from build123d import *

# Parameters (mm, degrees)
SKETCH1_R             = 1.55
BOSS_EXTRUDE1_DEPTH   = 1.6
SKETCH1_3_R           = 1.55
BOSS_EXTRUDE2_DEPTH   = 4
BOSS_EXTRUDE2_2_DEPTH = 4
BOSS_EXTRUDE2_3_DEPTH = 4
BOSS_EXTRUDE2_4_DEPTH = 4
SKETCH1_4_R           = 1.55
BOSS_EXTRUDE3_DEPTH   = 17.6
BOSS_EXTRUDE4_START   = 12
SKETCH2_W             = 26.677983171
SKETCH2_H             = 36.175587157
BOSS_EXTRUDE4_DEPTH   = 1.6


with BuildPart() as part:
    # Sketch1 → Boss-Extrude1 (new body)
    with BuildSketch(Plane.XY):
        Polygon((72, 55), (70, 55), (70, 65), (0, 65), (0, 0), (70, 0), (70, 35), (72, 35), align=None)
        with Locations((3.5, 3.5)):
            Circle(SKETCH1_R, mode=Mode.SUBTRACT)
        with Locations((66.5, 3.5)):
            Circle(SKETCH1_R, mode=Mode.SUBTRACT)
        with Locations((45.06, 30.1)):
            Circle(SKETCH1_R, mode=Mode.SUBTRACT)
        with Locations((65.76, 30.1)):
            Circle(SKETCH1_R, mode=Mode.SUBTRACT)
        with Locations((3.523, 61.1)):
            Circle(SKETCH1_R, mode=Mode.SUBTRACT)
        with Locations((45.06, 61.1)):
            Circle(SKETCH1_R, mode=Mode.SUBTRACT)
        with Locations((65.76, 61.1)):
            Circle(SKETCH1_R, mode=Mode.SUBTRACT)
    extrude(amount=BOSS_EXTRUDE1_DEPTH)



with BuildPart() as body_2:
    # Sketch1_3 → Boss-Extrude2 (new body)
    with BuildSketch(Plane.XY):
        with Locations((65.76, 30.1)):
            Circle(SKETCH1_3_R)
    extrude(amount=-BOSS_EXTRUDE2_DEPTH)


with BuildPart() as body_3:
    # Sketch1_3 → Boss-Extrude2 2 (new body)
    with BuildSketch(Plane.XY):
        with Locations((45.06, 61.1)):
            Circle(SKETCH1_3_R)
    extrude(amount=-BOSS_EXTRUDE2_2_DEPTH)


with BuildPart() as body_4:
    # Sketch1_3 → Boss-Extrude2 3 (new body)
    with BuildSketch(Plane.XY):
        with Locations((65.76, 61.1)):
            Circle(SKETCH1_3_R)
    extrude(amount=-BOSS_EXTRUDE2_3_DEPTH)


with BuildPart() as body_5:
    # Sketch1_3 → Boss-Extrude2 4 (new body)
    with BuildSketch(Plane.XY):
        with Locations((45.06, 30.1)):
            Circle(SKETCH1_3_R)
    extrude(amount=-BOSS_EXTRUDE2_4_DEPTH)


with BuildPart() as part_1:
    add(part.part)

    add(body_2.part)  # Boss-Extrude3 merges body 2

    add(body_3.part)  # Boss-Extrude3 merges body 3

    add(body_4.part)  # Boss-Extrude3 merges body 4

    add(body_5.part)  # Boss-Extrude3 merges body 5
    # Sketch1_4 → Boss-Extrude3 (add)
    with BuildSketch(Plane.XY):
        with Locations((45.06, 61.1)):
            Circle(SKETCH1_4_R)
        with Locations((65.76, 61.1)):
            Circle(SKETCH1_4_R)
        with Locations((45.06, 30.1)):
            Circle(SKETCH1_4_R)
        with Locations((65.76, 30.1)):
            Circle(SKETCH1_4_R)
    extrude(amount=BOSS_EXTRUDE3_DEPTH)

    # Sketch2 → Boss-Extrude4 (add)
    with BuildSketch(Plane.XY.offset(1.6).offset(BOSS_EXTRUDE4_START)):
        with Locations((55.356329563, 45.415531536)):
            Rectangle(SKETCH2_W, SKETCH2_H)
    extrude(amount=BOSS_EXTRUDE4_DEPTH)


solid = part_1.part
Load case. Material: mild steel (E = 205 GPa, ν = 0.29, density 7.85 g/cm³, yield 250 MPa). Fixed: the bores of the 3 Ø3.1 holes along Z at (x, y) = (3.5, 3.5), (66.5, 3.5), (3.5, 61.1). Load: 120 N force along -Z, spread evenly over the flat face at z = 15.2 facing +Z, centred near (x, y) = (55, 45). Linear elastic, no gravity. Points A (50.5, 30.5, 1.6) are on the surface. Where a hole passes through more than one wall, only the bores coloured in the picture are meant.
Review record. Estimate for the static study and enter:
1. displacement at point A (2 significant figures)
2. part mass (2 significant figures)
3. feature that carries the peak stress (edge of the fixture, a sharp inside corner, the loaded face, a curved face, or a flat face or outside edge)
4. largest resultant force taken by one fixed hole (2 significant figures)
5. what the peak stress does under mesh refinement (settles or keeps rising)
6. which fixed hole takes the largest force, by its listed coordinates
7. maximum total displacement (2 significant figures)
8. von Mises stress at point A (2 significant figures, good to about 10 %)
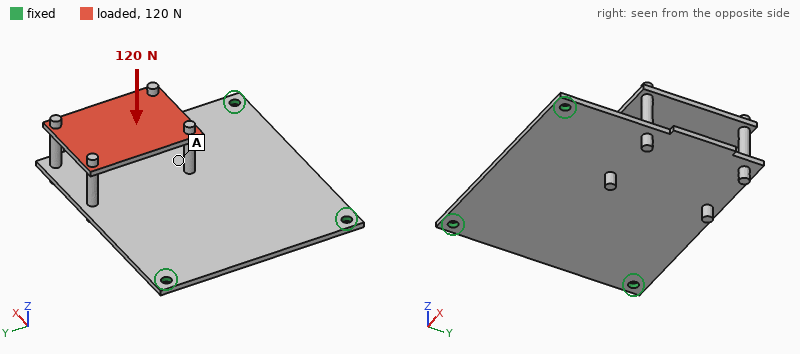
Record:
0.18 mm
74 g
edge of the fixture
81 N
keeps rising
(66.5, 3.5)
0.60 mm
27 MPa
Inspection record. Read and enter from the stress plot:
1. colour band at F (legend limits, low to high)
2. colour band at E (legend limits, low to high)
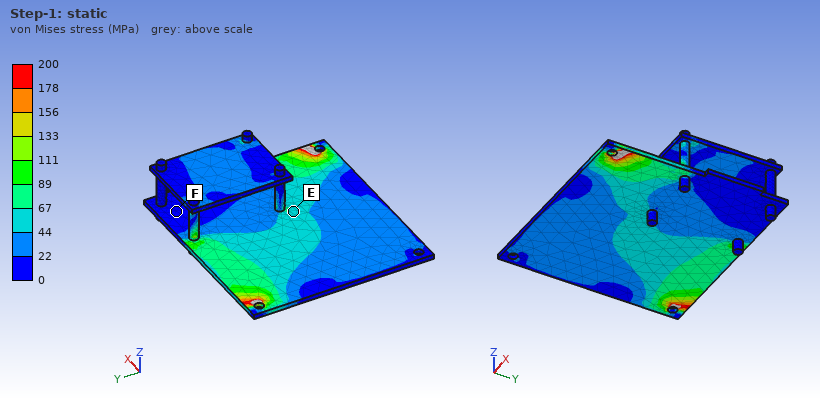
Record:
0 to 22 MPa
44 to 67 MPa
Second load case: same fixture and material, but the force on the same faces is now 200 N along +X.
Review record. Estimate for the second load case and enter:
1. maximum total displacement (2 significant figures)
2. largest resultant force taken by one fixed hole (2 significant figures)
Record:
0.34 mm
94 N
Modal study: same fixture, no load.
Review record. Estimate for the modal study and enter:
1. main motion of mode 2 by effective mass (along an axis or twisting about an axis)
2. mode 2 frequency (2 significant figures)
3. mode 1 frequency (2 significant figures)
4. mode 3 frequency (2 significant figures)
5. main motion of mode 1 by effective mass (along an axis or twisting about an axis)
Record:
along Z
1300 Hz
470 Hz
1700 Hz
along Z
